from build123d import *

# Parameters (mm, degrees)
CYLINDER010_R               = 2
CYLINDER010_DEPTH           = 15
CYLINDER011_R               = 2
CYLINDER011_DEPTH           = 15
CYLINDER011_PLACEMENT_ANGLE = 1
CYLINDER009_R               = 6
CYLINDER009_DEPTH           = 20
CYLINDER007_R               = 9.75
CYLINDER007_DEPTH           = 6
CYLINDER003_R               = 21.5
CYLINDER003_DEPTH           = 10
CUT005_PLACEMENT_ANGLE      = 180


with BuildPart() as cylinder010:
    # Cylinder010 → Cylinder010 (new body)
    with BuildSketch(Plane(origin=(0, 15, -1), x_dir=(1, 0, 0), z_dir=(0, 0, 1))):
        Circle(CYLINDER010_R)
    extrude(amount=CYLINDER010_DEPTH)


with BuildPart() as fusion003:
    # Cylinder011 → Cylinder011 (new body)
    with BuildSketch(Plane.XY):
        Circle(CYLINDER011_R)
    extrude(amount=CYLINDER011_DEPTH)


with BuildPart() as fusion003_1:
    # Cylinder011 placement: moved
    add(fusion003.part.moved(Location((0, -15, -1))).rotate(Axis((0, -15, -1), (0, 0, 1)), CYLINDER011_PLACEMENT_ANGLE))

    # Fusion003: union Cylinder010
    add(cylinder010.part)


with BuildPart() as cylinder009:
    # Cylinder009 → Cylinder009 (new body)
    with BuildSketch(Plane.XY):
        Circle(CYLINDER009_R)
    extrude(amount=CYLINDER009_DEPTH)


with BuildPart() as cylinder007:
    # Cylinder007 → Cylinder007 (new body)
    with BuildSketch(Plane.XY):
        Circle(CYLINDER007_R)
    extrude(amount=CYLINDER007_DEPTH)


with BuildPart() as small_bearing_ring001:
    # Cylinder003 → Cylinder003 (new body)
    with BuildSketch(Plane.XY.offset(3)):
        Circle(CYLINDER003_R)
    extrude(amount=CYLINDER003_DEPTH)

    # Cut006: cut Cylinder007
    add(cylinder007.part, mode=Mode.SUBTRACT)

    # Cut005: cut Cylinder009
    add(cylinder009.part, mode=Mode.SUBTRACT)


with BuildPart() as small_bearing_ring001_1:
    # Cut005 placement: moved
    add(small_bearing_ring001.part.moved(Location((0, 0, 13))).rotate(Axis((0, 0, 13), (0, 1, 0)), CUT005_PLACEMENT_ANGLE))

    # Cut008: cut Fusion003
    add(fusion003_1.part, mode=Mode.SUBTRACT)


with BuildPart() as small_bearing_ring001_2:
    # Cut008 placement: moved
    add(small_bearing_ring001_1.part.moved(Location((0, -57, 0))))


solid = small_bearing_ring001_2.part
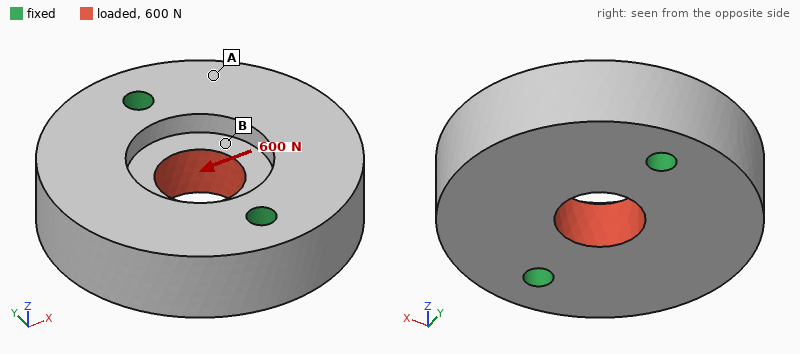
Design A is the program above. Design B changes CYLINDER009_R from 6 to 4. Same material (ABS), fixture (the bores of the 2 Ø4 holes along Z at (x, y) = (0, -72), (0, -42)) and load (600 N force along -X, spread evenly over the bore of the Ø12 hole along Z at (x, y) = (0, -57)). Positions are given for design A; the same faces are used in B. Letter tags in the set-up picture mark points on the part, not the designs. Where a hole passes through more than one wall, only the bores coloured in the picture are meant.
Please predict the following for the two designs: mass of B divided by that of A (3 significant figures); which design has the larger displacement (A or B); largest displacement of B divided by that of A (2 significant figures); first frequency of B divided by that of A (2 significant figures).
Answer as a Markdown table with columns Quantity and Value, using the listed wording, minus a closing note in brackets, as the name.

| Quantity | Value |
|---|---|
| mass of B divided by that of A | 1.03 |
| which design has the larger displacement | B |
| largest displacement of B divided by that of A | 1.1 |
| first frequency of B divided by that of A | 1.00 |
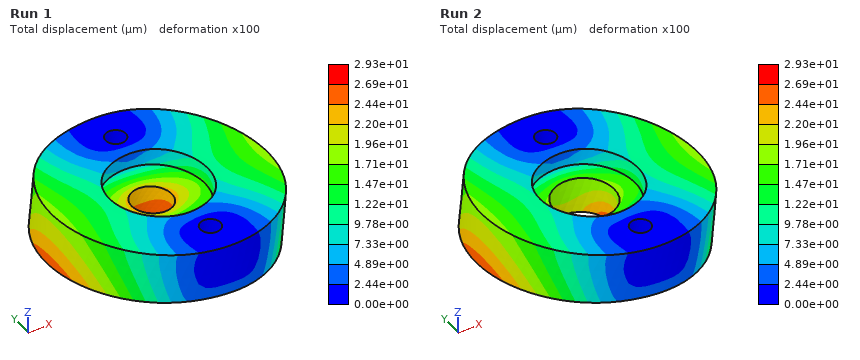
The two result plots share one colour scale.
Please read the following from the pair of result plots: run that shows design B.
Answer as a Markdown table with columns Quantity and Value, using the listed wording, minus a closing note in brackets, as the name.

| Quantity | Value |
|---|---|
| run that shows design B | Run 1 |
